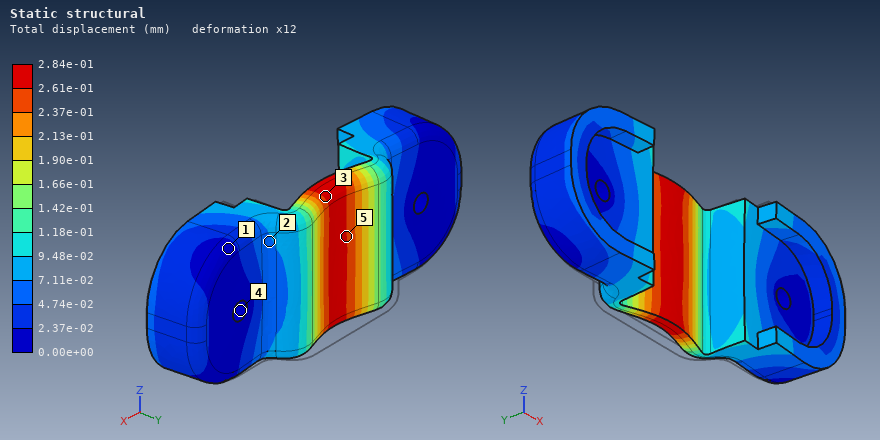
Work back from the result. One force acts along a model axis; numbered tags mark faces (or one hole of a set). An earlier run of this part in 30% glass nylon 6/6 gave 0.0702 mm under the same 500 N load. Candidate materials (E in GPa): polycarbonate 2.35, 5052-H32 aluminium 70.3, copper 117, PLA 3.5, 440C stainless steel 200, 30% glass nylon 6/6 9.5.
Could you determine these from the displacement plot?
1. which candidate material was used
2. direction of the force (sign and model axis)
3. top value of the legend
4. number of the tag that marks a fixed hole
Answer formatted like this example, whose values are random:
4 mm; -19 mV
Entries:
polycarbonate; -Y; 2.84e-01 mm; 4
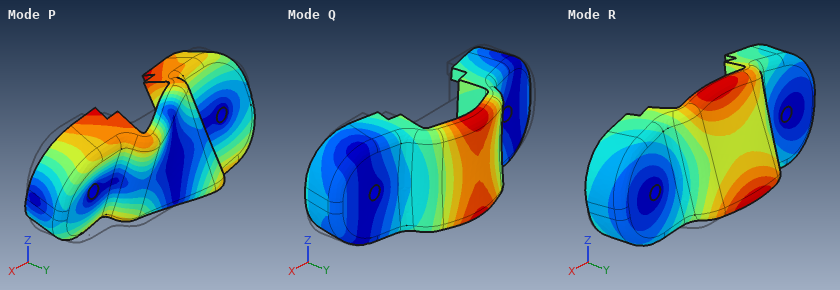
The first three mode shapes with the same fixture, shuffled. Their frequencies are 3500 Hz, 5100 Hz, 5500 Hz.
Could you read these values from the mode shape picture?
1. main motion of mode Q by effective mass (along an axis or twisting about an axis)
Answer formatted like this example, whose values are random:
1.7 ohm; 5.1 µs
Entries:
along Y
